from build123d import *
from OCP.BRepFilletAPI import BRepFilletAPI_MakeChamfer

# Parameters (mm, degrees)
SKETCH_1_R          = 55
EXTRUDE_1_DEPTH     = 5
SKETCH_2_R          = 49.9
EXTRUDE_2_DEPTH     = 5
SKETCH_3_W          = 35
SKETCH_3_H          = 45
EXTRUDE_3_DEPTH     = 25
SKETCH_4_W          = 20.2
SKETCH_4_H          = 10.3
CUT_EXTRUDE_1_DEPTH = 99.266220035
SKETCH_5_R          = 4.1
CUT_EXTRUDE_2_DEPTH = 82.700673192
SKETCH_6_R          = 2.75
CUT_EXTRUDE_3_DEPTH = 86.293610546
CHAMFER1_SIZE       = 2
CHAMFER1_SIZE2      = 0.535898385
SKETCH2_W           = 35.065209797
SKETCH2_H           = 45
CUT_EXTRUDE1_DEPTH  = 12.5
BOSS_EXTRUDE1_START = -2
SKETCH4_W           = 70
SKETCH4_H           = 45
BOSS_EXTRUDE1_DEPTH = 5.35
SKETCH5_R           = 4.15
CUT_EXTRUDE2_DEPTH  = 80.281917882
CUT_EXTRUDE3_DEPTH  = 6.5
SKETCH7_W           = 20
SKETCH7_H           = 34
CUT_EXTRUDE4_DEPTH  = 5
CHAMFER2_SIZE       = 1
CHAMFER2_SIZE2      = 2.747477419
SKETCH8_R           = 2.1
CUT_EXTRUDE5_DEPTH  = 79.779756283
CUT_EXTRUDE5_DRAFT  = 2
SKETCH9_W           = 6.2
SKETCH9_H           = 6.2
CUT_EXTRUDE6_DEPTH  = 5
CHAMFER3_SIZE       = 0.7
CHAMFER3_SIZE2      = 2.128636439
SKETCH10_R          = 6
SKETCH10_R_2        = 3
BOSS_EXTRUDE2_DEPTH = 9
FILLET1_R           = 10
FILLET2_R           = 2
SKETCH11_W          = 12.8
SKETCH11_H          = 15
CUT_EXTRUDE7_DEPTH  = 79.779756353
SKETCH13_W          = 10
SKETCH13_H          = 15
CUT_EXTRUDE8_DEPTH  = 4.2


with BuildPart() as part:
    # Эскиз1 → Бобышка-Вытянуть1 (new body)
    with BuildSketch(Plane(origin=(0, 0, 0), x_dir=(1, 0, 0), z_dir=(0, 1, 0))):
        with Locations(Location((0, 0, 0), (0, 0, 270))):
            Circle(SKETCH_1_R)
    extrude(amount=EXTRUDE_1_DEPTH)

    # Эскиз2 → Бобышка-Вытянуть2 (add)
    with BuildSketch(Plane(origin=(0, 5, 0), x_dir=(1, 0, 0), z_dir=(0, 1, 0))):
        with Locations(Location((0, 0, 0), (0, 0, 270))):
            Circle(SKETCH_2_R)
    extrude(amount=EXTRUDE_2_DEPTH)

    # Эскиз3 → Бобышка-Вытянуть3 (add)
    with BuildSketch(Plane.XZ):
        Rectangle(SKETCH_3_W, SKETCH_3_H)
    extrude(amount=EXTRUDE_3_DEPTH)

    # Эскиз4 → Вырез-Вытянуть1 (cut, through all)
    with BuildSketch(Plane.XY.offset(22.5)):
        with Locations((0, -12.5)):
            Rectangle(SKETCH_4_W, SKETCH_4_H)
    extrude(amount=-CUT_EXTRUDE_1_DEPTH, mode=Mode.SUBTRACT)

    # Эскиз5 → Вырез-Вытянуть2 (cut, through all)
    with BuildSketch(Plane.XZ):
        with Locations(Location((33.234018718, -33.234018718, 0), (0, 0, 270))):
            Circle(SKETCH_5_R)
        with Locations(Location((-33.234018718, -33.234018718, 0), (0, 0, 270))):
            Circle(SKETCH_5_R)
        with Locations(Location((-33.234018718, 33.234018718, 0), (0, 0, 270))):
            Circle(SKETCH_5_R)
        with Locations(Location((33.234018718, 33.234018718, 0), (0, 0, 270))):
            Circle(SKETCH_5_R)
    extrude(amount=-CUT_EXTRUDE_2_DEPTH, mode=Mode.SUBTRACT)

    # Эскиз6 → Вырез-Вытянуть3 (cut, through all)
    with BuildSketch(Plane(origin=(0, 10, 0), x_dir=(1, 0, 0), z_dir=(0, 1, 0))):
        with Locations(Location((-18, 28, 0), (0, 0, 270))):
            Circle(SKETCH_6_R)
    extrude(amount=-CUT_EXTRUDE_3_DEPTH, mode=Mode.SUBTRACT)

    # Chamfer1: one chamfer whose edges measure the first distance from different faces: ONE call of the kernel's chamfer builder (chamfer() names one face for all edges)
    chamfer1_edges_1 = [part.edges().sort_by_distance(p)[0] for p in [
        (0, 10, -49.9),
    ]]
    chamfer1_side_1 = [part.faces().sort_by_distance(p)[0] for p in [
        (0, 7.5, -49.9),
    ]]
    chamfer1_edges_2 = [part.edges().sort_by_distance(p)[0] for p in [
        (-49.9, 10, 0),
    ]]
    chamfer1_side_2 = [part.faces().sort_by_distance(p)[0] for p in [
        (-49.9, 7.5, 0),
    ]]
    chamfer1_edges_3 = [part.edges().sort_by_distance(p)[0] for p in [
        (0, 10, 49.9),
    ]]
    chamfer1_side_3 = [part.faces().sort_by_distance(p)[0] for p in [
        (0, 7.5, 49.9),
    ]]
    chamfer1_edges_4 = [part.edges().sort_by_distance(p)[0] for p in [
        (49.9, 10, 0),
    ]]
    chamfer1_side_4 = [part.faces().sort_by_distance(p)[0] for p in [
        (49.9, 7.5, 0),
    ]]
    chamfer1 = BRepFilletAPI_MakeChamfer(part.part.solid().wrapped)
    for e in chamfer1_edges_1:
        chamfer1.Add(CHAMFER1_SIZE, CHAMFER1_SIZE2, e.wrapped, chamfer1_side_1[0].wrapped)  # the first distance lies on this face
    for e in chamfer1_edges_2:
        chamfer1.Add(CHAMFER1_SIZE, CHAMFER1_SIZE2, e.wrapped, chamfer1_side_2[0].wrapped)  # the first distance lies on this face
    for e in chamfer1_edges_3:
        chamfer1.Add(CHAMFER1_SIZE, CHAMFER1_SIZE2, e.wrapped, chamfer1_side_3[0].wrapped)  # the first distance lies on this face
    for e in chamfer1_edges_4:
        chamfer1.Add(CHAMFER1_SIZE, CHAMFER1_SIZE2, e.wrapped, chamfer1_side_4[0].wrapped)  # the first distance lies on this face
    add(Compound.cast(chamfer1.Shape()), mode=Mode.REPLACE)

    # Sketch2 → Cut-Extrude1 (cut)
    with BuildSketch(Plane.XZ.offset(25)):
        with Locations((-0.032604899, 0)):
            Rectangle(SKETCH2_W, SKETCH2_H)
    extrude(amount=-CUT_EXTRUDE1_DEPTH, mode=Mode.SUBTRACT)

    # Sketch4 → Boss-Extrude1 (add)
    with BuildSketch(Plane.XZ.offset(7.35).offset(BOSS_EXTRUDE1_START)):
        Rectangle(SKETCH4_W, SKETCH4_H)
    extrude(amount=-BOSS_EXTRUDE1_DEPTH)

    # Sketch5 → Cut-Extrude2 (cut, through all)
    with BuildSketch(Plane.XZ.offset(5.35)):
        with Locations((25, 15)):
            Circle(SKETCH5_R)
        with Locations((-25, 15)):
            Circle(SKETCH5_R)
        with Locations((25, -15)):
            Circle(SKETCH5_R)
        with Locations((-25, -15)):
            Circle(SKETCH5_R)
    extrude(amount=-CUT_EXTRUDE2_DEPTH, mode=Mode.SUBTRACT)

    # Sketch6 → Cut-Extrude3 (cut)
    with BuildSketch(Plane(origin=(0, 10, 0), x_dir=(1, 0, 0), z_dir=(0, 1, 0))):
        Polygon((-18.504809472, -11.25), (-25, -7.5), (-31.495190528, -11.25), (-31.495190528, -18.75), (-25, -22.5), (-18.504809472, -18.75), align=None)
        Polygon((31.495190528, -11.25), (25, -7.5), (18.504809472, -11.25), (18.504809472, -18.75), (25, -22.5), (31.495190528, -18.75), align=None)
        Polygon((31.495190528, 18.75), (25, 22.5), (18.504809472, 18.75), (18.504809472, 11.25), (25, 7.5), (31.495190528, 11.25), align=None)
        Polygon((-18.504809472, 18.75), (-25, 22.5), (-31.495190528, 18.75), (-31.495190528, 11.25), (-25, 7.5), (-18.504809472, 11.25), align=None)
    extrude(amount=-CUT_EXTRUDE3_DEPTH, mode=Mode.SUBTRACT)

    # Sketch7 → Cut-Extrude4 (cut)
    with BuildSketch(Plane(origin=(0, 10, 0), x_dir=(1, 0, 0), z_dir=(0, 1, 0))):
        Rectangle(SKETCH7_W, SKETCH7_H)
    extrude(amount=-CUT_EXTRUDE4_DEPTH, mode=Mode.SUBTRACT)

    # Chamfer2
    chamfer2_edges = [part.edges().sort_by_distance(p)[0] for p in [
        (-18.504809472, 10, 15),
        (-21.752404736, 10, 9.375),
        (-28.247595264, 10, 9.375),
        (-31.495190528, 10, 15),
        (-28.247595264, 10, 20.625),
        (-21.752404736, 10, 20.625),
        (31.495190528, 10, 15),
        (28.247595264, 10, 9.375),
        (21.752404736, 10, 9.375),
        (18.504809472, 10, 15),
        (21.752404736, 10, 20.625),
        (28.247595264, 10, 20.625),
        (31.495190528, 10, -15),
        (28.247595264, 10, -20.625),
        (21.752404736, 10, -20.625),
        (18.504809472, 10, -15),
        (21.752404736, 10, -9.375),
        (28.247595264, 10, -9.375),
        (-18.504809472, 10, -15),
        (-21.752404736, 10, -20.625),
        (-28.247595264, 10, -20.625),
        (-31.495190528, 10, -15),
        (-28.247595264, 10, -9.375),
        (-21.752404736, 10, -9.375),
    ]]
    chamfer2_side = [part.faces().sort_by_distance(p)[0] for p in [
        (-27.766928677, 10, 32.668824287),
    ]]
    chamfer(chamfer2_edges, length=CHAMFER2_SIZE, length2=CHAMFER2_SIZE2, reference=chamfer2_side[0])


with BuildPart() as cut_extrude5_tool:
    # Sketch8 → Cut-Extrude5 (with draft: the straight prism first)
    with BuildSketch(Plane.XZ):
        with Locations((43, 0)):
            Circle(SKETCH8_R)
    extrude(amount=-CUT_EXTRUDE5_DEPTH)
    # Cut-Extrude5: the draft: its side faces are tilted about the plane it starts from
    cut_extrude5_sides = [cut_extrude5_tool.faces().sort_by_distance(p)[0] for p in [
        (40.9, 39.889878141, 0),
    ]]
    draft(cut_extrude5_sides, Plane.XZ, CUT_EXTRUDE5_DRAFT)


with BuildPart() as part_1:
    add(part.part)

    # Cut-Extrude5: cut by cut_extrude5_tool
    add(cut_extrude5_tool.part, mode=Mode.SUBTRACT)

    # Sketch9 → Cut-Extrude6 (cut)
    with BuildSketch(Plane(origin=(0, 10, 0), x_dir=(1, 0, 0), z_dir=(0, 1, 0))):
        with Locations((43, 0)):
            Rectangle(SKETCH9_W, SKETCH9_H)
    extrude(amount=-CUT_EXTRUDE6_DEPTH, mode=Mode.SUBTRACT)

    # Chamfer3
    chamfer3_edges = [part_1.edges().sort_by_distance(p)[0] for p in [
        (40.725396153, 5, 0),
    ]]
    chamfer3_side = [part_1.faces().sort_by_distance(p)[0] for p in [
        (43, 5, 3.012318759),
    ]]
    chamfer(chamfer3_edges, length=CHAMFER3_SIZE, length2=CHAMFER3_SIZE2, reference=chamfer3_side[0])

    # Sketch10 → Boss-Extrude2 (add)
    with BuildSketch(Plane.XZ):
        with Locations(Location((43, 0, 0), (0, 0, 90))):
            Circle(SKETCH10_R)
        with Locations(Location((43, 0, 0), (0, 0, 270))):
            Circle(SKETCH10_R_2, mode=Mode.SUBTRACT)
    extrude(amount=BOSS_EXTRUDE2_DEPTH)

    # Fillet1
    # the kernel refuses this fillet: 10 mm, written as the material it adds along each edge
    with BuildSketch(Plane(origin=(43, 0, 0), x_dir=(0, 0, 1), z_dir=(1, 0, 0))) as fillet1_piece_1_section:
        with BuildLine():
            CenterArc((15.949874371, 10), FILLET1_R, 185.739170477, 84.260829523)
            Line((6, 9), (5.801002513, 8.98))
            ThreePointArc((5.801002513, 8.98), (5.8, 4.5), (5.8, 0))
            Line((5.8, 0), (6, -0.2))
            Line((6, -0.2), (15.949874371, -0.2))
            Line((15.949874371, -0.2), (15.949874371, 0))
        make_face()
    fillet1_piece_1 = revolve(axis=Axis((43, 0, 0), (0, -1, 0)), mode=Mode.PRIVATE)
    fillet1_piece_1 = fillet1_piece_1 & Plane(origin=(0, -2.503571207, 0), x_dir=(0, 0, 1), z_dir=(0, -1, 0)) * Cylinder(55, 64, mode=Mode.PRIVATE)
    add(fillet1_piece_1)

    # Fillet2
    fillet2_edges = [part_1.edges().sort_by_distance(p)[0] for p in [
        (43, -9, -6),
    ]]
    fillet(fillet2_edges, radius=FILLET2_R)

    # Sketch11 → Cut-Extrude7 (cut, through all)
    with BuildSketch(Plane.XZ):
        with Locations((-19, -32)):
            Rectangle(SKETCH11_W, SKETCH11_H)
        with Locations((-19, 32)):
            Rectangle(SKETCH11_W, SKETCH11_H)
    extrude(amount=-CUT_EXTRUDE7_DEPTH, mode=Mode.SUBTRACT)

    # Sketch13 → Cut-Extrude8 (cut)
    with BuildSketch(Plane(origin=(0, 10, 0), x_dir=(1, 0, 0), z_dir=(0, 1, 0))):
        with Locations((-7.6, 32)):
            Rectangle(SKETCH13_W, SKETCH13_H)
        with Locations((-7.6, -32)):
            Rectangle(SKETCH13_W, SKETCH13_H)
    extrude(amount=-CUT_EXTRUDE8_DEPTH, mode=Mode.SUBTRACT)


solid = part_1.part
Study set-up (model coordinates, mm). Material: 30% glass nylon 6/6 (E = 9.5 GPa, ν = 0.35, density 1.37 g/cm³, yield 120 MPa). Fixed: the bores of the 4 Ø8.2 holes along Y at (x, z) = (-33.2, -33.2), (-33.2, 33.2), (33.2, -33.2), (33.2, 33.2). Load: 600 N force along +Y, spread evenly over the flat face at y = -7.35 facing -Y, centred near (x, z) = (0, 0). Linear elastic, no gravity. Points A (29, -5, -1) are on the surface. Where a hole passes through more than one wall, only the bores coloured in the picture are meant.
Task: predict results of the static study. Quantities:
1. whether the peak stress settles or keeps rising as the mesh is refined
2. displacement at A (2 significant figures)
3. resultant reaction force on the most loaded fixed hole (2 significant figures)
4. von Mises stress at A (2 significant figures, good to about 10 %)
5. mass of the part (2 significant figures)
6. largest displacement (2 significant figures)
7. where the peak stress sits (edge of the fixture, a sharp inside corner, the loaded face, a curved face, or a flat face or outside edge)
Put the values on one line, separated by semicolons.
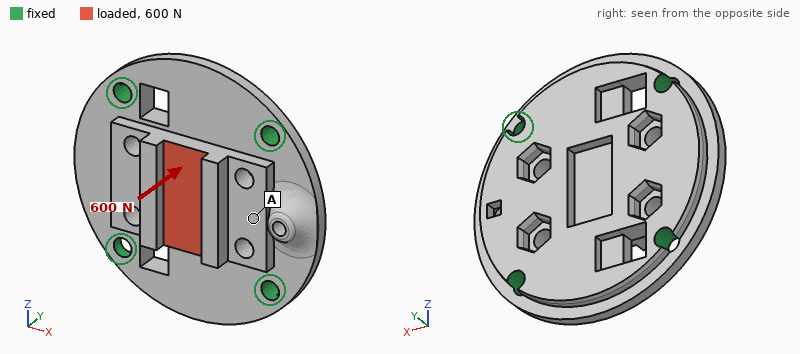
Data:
keeps rising; 9.2 µm; 190 N; 0.88 MPa; 130 g; 22 µm; edge of the fixture
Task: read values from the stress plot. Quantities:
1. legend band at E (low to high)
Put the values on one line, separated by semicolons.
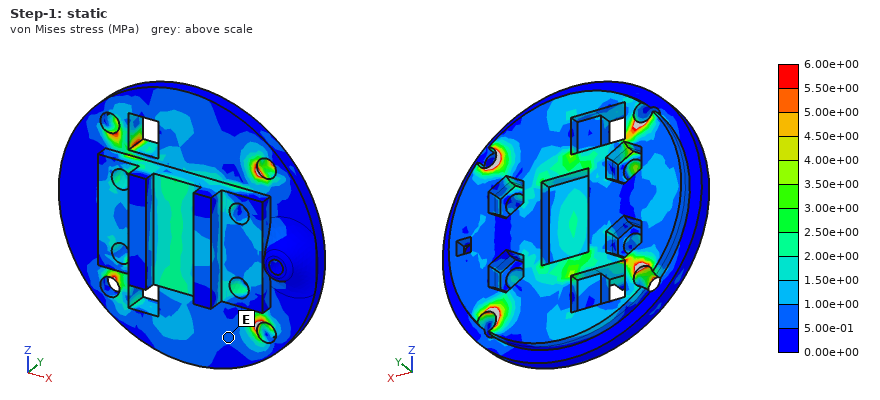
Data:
5.00e-01 to 1.00e+00 MPa
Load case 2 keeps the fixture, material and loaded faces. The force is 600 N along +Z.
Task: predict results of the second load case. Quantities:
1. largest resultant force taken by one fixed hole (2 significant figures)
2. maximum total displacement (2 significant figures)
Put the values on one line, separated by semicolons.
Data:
210 N; 9.8 µm
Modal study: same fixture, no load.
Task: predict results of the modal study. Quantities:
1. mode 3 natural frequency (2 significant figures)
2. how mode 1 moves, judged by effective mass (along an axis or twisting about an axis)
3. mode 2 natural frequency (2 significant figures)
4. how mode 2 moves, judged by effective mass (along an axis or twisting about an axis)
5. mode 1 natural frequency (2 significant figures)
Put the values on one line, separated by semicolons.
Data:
4800 Hz; along Y; 4600 Hz; twisting about X; 3800 Hz
